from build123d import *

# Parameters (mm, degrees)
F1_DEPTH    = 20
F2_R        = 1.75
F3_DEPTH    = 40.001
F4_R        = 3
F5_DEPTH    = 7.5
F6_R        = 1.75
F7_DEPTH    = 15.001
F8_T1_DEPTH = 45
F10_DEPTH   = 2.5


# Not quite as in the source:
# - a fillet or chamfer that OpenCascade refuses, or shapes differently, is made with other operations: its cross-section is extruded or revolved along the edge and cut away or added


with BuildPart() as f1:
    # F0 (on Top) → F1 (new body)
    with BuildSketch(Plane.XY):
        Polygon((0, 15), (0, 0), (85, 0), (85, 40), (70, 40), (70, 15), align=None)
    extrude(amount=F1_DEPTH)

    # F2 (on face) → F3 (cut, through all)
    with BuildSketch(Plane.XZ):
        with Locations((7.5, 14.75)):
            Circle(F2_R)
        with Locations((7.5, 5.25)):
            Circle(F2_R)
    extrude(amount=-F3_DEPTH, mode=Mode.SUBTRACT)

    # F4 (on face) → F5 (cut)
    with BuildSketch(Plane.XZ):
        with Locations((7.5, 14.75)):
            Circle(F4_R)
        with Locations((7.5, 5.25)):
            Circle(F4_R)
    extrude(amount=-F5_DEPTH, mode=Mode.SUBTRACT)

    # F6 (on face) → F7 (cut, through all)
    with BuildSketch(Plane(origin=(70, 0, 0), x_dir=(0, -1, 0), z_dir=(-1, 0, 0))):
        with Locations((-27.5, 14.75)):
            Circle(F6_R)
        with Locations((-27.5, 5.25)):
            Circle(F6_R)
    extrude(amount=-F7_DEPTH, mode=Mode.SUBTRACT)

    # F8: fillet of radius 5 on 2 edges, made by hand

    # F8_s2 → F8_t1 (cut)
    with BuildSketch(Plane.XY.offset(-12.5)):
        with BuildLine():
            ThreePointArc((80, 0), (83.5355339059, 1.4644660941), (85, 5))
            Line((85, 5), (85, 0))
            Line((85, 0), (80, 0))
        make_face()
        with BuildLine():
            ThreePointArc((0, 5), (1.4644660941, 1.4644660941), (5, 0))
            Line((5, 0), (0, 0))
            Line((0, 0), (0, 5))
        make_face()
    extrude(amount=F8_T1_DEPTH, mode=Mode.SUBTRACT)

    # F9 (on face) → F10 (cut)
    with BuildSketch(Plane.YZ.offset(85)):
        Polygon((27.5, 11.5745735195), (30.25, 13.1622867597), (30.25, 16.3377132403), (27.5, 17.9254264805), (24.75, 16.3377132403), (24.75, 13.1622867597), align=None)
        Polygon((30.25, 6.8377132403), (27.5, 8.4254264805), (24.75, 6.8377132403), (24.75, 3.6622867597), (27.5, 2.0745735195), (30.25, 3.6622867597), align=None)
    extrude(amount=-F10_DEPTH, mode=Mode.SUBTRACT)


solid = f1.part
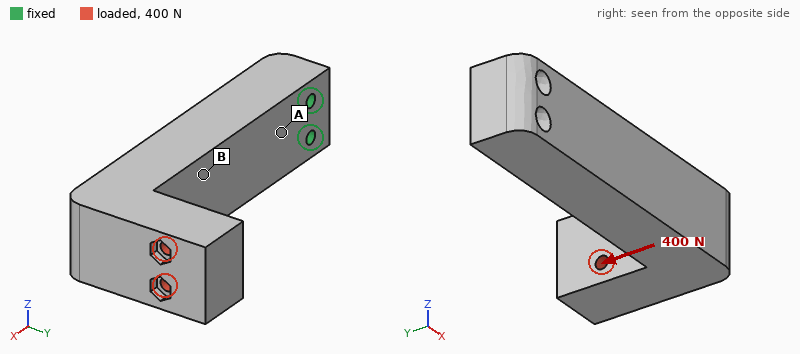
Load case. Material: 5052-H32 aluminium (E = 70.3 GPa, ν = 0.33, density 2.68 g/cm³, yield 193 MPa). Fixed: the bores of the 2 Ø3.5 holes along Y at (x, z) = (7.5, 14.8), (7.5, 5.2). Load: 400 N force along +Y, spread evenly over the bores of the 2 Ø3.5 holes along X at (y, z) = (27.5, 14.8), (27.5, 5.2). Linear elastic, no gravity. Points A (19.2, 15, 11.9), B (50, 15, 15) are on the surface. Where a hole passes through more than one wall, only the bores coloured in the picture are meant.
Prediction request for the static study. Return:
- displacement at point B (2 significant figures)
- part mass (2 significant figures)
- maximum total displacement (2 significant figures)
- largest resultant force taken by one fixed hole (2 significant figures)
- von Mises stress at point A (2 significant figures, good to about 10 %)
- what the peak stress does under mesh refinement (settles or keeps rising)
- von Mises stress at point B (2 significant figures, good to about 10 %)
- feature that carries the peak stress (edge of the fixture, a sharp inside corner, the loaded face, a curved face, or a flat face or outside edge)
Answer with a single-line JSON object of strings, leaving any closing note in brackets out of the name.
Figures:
{"displacement at point B": "0.10 mm", "part mass": "85 g", "maximum total displacement": "0.25 mm", "largest resultant force taken by one fixed hole": "250 N", "von Mises stress at point A": "33 MPa", "what the peak stress does under mesh refinement": "keeps rising", "von Mises stress at point B": "14 MPa", "feature that carries the peak stress": "edge of the fixture"}
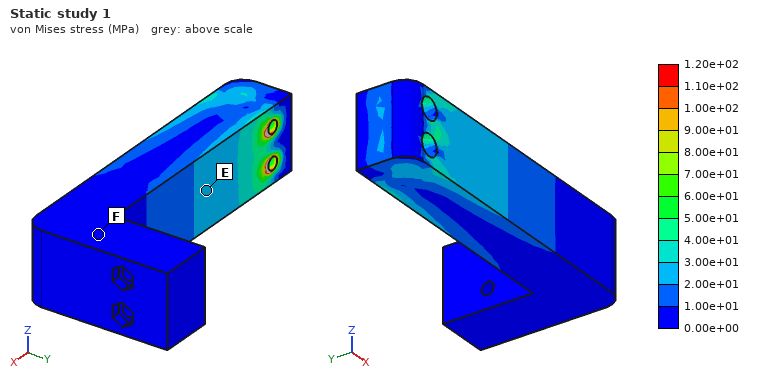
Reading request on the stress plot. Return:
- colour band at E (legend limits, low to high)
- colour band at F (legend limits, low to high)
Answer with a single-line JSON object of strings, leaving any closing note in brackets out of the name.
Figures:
{"colour band at E": "2.00e+01 to 3.00e+01 MPa", "colour band at F": "0.00e+00 to 1.00e+01 MPa"}
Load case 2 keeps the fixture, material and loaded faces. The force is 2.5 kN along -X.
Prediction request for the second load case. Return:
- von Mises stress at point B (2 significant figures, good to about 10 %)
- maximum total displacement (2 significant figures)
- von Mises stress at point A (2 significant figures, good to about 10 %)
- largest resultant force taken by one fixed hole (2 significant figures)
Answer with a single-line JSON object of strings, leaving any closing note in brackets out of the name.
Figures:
{"von Mises stress at point B": "75 MPa", "maximum total displacement": "0.62 mm", "von Mises stress at point A": "79 MPa", "largest resultant force taken by one fixed hole": "1.3 kN"}
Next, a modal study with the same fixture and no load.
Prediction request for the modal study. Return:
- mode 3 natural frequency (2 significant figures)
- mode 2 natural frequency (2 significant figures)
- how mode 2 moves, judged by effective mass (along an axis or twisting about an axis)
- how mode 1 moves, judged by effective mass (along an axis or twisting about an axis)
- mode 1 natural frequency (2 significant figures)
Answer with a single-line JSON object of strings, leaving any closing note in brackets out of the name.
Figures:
{"mode 3 natural frequency": "4100 Hz", "mode 2 natural frequency": "1600 Hz", "how mode 2 moves, judged by effective mass": "along Z", "how mode 1 moves, judged by effective mass": "along Y", "mode 1 natural frequency": "1100 Hz"}
